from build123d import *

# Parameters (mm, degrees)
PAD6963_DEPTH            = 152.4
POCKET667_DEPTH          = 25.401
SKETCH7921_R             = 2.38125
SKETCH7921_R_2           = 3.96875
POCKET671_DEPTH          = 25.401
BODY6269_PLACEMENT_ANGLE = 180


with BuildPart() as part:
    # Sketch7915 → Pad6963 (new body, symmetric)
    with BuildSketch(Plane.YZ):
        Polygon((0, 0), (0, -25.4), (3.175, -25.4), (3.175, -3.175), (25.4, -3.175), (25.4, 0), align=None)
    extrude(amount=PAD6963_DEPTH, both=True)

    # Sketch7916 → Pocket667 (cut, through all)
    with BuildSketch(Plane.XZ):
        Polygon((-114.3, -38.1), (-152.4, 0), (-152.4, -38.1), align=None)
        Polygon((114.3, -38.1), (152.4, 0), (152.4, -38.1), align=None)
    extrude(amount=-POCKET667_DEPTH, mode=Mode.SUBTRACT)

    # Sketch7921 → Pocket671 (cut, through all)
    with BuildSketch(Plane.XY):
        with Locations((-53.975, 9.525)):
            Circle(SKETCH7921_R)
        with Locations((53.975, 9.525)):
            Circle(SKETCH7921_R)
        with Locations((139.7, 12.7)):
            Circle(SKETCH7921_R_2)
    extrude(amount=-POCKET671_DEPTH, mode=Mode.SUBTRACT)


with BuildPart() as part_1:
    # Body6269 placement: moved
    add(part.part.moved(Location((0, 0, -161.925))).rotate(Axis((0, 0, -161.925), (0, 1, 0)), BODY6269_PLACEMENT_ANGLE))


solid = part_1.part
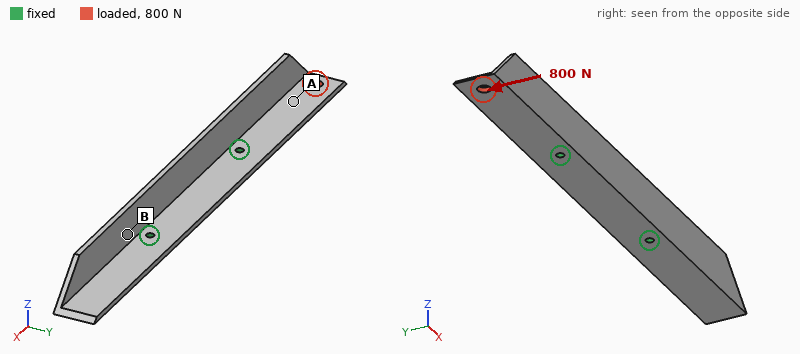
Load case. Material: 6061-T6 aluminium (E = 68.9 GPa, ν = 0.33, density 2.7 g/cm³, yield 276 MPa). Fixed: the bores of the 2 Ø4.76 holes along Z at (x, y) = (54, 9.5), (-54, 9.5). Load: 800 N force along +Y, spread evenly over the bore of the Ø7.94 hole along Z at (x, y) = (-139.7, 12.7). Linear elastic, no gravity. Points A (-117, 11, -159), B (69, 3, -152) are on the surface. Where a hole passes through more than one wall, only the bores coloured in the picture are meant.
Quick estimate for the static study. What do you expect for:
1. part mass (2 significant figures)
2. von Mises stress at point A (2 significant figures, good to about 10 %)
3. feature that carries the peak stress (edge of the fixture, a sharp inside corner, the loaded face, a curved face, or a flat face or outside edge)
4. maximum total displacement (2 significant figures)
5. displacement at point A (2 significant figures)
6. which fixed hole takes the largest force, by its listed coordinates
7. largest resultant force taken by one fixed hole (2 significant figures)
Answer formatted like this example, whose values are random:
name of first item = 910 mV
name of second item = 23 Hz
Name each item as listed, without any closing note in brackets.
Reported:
part mass = 120 g
von Mises stress at point A = 23 MPa
feature that carries the peak stress = edge of the fixture
maximum total displacement = 1.0 mm
displacement at point A = 0.57 mm
which fixed hole takes the largest force, by its listed coordinates = (-54, 9.5)
largest resultant force taken by one fixed hole = 1.3 kN
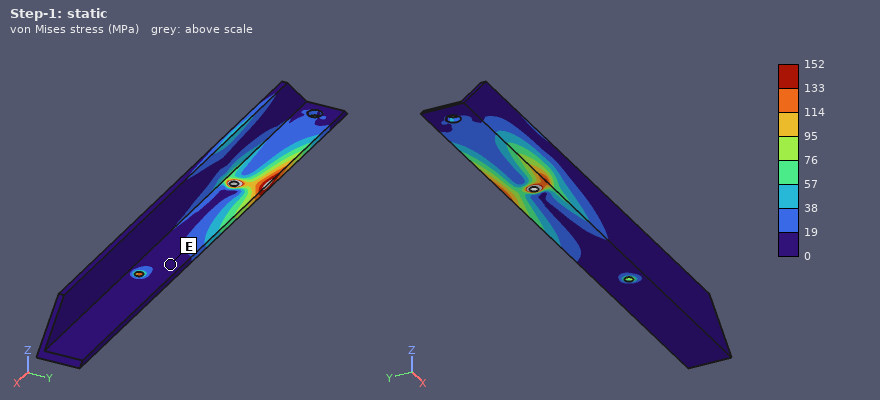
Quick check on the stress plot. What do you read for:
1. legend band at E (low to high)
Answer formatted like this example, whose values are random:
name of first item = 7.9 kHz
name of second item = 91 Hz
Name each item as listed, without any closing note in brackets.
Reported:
legend band at E = 0 to 19 MPa
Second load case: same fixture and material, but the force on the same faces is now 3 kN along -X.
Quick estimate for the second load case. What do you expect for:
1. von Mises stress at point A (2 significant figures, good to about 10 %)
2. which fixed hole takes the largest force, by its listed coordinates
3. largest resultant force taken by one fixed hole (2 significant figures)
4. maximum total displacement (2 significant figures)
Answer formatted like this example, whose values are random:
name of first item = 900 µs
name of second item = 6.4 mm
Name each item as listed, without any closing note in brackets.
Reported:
von Mises stress at point A = 30 MPa
which fixed hole takes the largest force, by its listed coordinates = (-54, 9.5)
largest resultant force taken by one fixed hole = 2.7 kN
maximum total displacement = 0.15 mm
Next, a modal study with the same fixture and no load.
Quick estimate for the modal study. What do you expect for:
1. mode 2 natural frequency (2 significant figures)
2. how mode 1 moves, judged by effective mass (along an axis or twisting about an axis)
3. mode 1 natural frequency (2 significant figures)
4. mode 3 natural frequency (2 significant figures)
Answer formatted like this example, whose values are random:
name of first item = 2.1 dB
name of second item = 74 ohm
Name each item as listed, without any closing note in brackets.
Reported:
mode 2 natural frequency = 1100 Hz
how mode 1 moves, judged by effective mass = along Z
mode 1 natural frequency = 1100 Hz
mode 3 natural frequency = 1100 Hz
